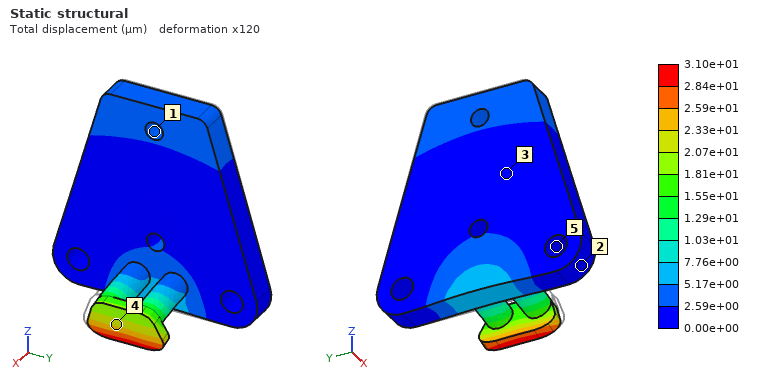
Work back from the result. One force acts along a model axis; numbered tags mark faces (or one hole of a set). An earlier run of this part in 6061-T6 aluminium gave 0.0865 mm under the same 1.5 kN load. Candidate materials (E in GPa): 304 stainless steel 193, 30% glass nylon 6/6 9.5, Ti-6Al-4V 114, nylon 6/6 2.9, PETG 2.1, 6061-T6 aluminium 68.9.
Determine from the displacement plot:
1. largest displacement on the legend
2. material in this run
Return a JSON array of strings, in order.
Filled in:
["3.10e+01 µm", "304 stainless steel"]
